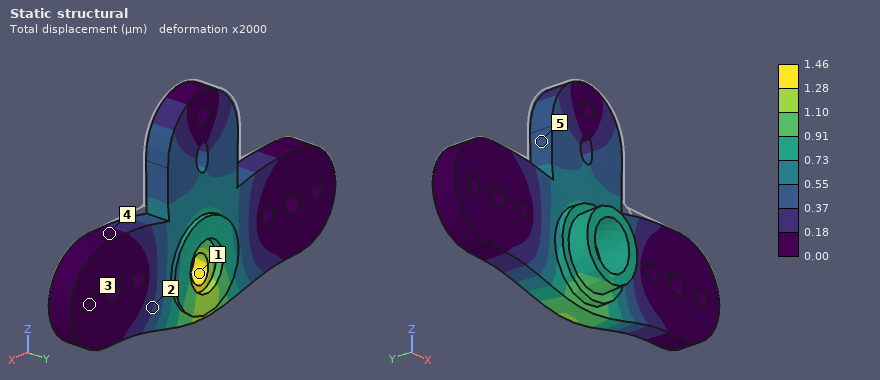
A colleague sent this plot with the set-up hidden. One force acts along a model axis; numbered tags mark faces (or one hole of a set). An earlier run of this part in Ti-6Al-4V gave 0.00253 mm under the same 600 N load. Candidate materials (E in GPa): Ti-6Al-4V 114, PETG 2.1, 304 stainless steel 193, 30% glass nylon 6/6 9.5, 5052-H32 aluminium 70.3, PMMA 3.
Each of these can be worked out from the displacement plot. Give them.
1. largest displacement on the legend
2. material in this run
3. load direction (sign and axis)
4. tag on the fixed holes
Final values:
1.46 µm
304 stainless steel
-Z
3
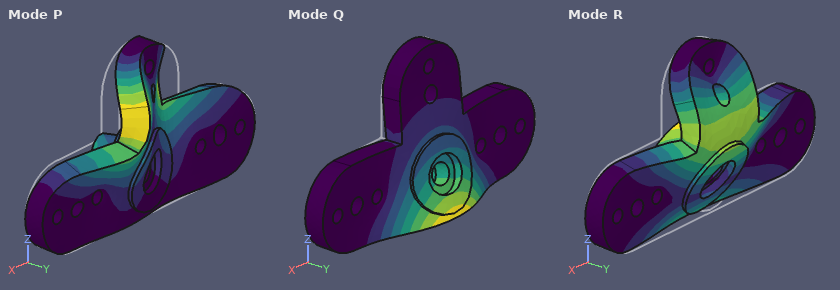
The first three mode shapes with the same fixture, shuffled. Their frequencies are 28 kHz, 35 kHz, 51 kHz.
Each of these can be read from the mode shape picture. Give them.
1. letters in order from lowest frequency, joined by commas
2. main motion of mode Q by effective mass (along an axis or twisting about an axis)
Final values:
Q, R, P
along Y
